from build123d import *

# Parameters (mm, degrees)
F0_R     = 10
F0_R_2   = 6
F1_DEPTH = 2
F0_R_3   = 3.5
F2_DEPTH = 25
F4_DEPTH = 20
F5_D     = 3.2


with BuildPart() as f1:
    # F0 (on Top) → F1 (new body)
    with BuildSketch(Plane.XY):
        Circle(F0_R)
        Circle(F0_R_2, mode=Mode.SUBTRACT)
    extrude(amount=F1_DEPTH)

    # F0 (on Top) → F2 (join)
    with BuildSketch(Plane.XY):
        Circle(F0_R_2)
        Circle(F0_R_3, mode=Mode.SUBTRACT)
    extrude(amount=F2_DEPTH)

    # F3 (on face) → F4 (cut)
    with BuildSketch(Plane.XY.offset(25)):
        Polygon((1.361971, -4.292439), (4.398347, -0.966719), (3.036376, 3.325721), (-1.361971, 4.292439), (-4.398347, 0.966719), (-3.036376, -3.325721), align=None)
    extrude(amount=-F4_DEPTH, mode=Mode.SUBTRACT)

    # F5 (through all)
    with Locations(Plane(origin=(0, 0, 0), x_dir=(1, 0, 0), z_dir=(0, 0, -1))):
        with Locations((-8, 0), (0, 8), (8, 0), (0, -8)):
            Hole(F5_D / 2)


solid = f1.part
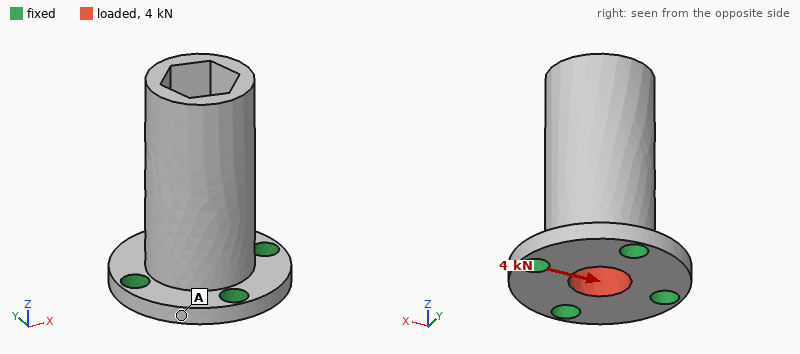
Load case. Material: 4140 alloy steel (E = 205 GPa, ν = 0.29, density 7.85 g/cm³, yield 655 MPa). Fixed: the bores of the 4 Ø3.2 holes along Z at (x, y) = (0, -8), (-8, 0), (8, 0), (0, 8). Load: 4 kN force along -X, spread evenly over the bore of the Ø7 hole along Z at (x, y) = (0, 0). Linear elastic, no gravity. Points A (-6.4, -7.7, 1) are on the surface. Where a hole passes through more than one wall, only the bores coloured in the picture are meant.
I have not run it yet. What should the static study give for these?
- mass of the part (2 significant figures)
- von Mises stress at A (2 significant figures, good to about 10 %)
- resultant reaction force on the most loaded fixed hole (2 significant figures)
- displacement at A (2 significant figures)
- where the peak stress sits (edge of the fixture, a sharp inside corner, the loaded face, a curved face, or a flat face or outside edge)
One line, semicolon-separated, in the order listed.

15 g; 30 MPa; 1.3 kN; 1.1 µm; edge of the fixture
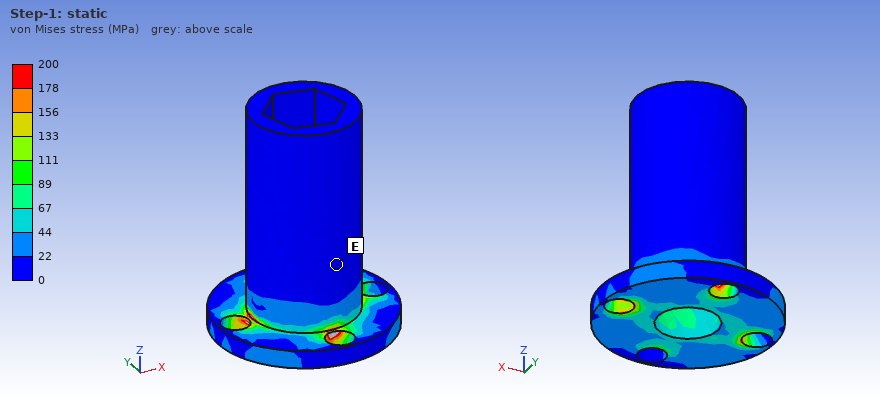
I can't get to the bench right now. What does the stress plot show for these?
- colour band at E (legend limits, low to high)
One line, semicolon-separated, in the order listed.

0 to 22 MPa
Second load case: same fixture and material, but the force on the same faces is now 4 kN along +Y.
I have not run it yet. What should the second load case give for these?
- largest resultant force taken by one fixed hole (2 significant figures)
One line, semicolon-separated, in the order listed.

1.3 kN
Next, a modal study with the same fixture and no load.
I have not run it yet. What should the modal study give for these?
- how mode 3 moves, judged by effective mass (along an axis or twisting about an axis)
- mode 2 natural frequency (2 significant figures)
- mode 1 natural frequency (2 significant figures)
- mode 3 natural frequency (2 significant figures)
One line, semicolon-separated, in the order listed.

twisting about Z; 12 kHz; 12 kHz; 33 kHz
